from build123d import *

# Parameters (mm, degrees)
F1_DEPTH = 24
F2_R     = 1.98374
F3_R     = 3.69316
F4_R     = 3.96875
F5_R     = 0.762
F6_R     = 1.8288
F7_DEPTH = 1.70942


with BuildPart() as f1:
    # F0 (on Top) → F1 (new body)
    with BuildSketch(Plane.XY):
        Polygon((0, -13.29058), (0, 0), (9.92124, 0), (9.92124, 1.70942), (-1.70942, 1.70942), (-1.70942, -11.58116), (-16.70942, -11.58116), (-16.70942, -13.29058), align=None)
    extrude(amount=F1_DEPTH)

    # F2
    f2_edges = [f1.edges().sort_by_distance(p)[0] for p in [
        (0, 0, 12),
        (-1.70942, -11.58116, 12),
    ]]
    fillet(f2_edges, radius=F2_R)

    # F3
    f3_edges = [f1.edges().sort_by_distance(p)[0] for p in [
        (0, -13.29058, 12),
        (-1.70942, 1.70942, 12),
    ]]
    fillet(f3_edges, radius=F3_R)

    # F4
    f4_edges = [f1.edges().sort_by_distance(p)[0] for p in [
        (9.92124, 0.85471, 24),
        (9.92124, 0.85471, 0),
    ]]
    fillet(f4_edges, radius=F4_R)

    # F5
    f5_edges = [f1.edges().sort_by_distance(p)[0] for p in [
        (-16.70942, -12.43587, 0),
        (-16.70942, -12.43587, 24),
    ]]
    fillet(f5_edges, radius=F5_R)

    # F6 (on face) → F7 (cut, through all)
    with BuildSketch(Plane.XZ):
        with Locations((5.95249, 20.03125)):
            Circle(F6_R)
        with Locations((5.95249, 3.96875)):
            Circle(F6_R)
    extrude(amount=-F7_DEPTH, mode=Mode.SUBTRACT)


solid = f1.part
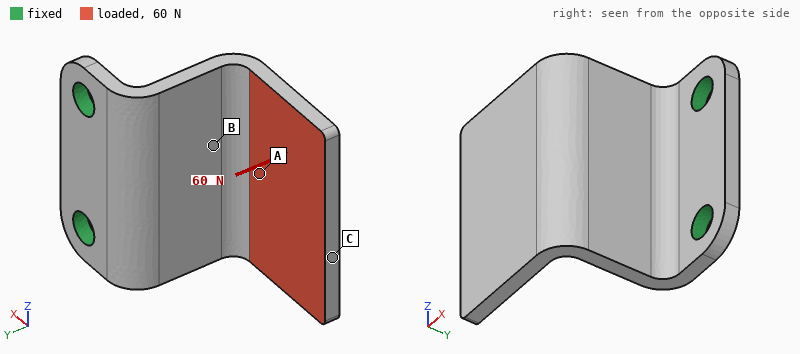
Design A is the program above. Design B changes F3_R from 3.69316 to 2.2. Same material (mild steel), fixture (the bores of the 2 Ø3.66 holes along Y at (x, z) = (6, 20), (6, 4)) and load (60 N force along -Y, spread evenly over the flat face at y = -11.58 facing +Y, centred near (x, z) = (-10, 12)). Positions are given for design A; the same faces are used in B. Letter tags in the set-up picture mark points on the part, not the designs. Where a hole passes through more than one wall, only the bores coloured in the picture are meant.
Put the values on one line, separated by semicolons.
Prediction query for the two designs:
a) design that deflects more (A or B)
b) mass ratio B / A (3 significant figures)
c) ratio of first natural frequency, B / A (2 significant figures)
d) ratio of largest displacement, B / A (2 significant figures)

A; 1.06; 1.0; 0.90
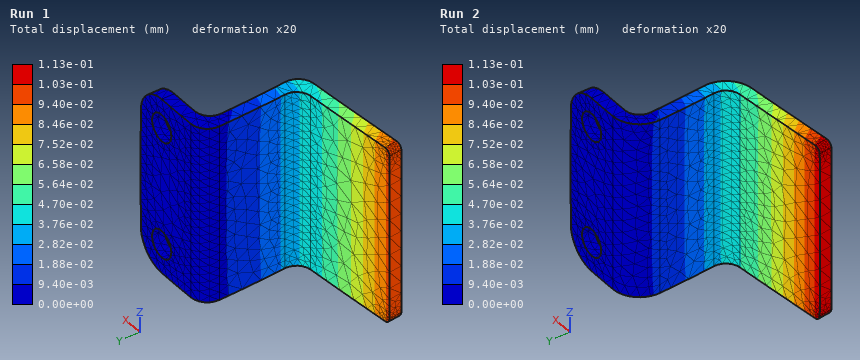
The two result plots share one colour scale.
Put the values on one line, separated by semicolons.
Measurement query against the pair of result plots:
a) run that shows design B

Run 1
